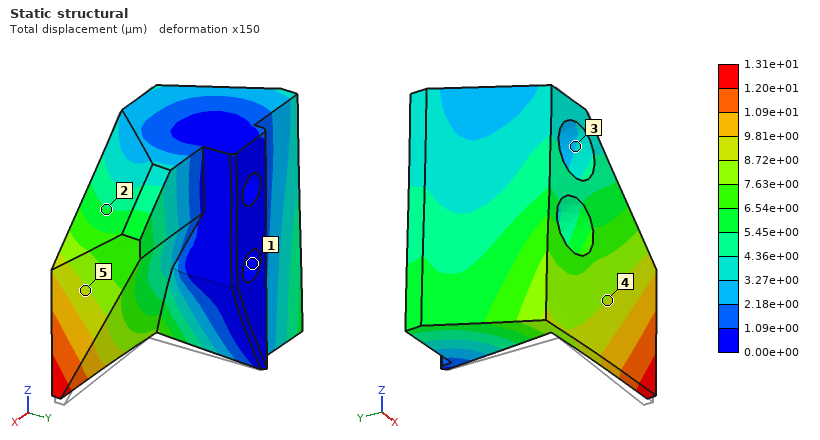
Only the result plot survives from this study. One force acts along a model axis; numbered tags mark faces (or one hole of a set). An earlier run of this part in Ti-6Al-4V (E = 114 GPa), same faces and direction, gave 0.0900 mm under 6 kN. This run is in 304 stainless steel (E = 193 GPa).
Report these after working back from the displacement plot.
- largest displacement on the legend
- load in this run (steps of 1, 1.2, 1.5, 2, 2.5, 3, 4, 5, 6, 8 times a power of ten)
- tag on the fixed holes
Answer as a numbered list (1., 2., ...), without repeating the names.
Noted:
1. 1.31e+01 µm
2. 1.5 kN
3. 1
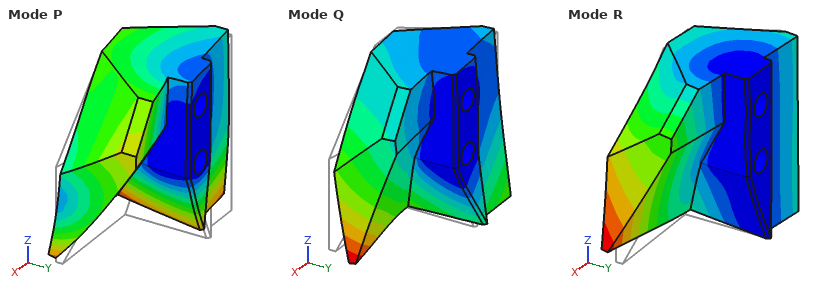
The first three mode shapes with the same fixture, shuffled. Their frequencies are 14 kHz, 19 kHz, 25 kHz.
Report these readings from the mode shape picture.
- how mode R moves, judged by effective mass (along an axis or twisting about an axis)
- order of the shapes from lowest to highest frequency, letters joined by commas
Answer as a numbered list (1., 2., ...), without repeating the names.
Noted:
1. along X
2. R, Q, P
